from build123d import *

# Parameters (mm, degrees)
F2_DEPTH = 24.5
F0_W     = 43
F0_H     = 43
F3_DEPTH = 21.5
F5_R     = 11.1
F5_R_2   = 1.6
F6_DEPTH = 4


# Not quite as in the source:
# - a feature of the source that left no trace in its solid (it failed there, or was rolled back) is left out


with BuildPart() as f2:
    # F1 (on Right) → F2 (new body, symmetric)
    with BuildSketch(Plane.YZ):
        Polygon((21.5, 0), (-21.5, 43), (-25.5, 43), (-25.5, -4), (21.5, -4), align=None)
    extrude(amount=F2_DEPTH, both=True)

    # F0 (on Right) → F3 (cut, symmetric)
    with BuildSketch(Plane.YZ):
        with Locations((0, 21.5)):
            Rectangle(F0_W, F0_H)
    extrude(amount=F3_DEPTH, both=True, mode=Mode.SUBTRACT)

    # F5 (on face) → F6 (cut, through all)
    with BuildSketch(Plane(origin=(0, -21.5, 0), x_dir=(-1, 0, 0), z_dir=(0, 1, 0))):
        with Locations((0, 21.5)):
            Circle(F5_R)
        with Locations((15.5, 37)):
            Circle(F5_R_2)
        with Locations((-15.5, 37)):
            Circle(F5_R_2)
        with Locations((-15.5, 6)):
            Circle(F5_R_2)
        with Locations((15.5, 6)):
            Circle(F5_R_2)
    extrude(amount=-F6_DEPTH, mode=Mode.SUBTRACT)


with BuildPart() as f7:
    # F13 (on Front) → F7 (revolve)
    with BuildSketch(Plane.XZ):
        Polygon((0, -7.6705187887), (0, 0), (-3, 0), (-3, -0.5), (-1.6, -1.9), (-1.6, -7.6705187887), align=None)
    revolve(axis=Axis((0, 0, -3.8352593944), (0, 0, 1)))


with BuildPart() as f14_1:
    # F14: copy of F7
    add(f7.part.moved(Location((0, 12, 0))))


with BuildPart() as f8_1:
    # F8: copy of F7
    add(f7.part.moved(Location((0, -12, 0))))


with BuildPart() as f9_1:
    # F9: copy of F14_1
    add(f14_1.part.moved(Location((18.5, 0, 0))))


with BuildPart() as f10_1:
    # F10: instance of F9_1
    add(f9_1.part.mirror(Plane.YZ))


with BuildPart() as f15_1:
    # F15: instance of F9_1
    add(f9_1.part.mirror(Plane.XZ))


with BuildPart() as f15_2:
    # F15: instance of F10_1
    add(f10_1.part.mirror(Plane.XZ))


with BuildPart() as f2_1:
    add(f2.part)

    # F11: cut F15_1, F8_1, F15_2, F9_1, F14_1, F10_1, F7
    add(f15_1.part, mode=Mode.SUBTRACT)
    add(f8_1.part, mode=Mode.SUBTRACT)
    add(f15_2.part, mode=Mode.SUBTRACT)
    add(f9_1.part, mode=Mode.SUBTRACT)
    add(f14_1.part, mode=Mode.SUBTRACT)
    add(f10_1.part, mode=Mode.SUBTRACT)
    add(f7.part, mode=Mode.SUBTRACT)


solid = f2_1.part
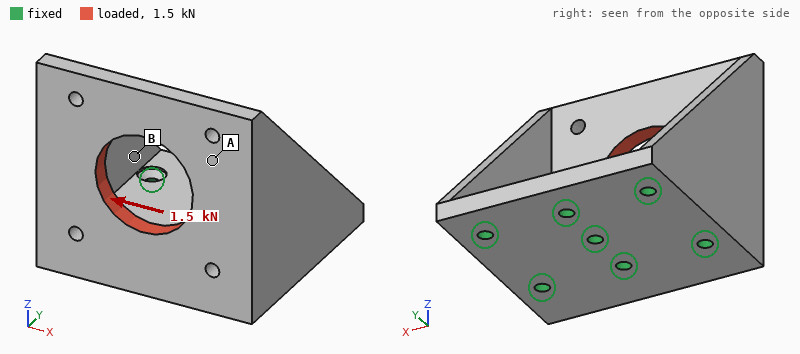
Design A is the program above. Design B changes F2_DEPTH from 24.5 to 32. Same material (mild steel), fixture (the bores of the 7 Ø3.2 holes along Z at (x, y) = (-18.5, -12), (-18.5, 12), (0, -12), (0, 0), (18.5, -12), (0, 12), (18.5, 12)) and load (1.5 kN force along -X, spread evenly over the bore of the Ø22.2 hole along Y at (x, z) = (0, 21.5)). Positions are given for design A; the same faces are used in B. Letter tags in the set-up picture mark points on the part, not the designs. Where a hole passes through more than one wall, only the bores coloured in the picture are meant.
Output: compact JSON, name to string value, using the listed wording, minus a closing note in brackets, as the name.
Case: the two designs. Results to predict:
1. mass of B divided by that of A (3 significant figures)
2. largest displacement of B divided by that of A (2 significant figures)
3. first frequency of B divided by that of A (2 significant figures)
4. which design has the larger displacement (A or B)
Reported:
{"mass of B divided by that of A": "1.91", "largest displacement of B divided by that of A": "0.80", "first frequency of B divided by that of A": "0.78", "which design has the larger displacement": "A"}
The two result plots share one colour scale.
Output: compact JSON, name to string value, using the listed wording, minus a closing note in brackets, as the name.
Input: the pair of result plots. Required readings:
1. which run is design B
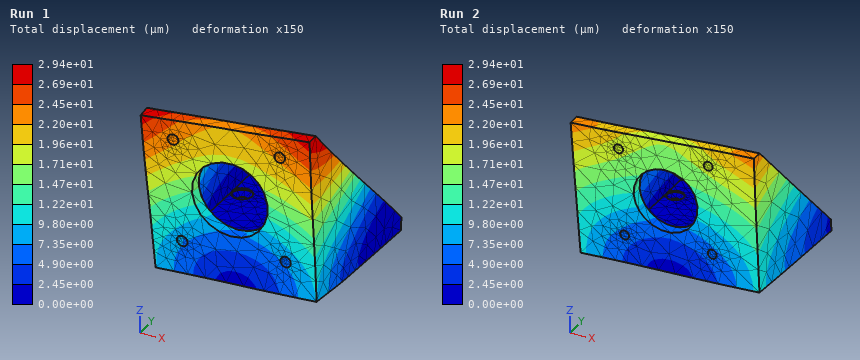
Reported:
{"which run is design B": "Run 2"}
